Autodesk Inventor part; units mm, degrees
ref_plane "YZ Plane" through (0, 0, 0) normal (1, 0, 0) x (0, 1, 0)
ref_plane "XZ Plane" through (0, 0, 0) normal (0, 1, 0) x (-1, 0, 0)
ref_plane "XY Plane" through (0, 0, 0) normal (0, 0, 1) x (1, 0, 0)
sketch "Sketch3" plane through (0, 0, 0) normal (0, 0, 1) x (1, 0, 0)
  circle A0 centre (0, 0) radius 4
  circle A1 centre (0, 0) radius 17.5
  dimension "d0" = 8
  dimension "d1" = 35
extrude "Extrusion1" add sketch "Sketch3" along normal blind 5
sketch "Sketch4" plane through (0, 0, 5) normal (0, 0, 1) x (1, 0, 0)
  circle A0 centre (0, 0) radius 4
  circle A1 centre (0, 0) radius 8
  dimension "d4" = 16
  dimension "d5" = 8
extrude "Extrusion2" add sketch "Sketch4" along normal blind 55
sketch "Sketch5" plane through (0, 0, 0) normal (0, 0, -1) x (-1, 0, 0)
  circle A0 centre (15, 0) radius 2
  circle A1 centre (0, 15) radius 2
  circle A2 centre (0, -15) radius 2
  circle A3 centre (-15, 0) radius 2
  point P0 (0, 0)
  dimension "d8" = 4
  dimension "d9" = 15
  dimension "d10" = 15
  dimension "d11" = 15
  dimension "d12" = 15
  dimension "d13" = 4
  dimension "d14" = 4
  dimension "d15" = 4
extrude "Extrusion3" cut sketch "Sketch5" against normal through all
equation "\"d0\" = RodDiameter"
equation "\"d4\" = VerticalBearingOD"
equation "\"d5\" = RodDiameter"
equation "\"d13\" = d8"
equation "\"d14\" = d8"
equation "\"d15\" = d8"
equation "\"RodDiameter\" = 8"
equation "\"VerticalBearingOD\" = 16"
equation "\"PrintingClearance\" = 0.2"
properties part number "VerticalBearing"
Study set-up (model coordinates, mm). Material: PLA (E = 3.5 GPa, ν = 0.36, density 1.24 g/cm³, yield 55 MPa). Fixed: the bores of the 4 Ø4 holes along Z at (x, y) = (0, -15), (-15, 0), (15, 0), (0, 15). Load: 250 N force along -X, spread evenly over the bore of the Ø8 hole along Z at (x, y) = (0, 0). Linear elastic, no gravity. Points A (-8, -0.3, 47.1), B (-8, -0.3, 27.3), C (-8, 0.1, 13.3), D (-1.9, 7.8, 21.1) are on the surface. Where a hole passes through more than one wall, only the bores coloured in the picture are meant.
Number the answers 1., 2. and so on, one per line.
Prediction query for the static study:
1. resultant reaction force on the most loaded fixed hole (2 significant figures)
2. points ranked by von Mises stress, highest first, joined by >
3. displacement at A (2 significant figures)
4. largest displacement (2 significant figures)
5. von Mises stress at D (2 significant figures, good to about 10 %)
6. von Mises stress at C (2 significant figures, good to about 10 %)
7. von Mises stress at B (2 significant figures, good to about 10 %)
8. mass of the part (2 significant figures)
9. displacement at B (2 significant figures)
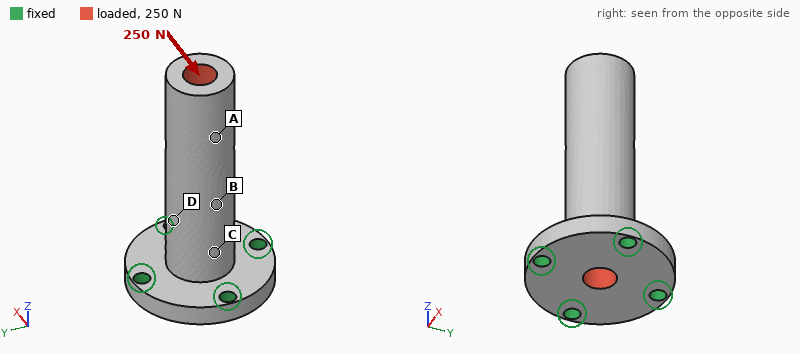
1. 280 N
2. C > B > D > A
3. 0.64 mm
4. 0.86 mm
5. 3.5 MPa
6. 12 MPa
7. 5.9 MPa
8. 16 g
9. 0.32 mm
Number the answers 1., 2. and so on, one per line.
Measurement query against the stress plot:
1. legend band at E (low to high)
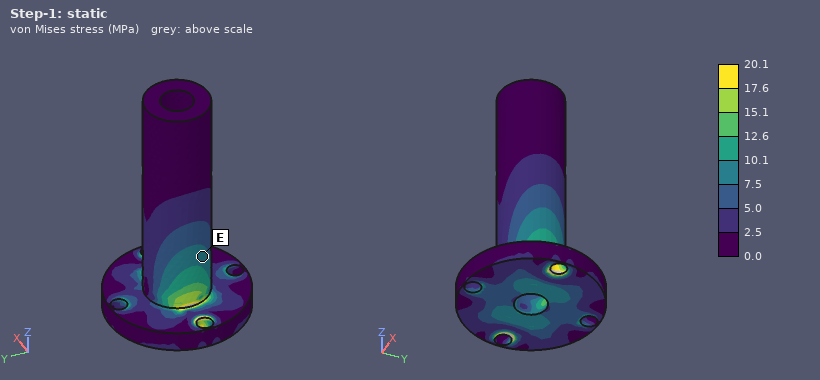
1. 7.5 to 10.1 MPa
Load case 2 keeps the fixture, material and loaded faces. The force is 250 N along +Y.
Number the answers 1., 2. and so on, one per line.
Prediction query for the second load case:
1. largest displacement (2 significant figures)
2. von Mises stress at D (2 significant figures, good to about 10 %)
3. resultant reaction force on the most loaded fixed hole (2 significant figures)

1. 0.86 mm
2. 8.1 MPa
3. 280 N
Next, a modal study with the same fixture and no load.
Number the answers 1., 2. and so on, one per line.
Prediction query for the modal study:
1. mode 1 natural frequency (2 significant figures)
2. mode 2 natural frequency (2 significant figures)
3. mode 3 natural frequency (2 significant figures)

1. 990 Hz
2. 990 Hz
3. 4400 Hz
